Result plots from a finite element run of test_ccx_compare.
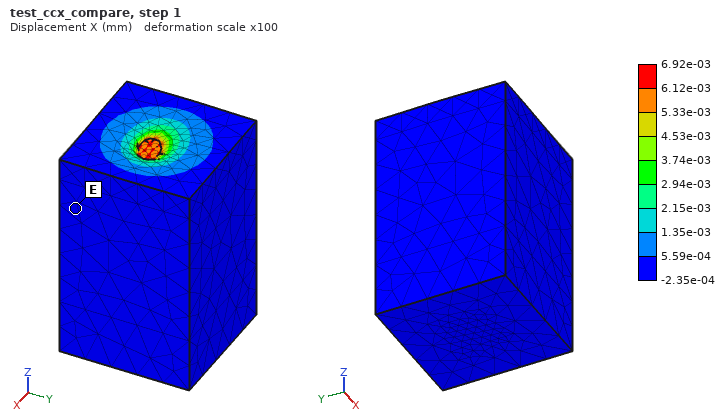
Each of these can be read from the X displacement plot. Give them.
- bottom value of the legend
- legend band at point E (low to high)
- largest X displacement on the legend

-2.35e-04 mm
-2.35e-04 to 5.59e-04 mm
6.92e-03 mm
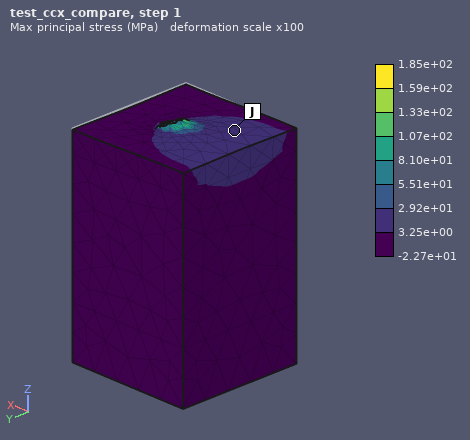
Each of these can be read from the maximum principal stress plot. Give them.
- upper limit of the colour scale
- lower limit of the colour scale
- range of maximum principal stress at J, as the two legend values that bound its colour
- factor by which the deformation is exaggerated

1.85e+02 MPa
-2.27e+01 MPa
3.25e+00 to 2.92e+01 MPa
100
